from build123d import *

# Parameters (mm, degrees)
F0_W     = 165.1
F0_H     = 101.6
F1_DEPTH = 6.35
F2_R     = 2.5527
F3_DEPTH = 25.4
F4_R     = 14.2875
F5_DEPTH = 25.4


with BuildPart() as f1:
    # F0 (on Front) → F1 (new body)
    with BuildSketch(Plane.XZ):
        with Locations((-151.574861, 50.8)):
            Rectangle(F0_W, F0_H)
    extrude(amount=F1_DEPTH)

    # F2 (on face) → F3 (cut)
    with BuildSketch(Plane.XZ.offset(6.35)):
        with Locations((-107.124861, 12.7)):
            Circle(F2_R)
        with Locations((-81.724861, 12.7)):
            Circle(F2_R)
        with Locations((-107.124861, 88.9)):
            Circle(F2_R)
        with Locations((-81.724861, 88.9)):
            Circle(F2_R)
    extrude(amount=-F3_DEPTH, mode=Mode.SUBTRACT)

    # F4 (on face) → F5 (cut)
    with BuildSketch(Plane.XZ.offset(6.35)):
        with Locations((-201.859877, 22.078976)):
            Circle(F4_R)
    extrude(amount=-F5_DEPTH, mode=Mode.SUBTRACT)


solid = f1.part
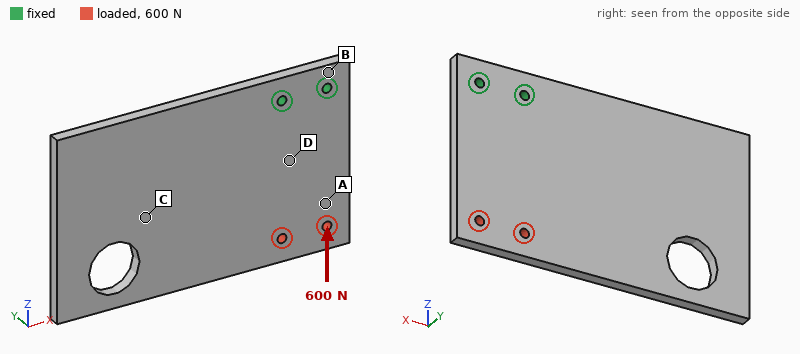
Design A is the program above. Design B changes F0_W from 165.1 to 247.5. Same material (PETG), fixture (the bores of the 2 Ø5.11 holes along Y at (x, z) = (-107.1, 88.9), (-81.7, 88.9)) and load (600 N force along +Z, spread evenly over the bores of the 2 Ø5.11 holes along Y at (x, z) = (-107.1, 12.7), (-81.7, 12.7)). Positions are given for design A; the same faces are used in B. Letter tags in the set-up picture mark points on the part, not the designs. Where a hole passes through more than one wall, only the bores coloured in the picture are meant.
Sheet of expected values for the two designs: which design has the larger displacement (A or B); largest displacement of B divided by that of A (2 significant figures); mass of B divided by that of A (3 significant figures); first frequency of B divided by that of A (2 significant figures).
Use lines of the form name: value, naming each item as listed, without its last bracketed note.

which design has the larger displacement: A
largest displacement of B divided by that of A: 0.84
mass of B divided by that of A: 1.52
first frequency of B divided by that of A: 0.61
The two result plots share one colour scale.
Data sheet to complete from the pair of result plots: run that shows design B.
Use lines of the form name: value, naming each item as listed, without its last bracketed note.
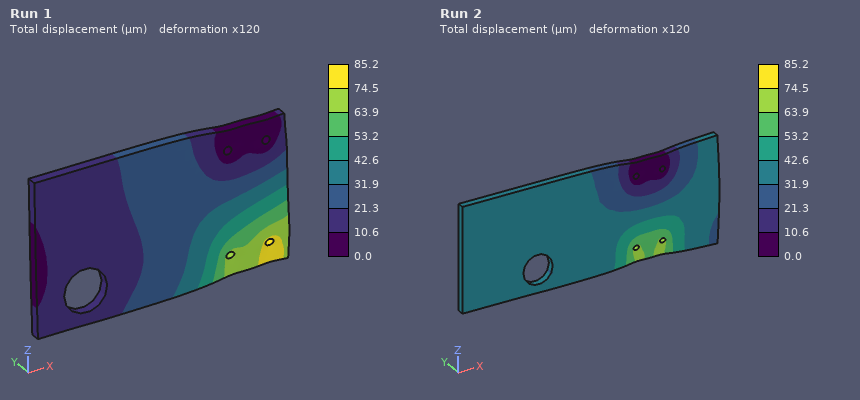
run that shows design B: Run 2
